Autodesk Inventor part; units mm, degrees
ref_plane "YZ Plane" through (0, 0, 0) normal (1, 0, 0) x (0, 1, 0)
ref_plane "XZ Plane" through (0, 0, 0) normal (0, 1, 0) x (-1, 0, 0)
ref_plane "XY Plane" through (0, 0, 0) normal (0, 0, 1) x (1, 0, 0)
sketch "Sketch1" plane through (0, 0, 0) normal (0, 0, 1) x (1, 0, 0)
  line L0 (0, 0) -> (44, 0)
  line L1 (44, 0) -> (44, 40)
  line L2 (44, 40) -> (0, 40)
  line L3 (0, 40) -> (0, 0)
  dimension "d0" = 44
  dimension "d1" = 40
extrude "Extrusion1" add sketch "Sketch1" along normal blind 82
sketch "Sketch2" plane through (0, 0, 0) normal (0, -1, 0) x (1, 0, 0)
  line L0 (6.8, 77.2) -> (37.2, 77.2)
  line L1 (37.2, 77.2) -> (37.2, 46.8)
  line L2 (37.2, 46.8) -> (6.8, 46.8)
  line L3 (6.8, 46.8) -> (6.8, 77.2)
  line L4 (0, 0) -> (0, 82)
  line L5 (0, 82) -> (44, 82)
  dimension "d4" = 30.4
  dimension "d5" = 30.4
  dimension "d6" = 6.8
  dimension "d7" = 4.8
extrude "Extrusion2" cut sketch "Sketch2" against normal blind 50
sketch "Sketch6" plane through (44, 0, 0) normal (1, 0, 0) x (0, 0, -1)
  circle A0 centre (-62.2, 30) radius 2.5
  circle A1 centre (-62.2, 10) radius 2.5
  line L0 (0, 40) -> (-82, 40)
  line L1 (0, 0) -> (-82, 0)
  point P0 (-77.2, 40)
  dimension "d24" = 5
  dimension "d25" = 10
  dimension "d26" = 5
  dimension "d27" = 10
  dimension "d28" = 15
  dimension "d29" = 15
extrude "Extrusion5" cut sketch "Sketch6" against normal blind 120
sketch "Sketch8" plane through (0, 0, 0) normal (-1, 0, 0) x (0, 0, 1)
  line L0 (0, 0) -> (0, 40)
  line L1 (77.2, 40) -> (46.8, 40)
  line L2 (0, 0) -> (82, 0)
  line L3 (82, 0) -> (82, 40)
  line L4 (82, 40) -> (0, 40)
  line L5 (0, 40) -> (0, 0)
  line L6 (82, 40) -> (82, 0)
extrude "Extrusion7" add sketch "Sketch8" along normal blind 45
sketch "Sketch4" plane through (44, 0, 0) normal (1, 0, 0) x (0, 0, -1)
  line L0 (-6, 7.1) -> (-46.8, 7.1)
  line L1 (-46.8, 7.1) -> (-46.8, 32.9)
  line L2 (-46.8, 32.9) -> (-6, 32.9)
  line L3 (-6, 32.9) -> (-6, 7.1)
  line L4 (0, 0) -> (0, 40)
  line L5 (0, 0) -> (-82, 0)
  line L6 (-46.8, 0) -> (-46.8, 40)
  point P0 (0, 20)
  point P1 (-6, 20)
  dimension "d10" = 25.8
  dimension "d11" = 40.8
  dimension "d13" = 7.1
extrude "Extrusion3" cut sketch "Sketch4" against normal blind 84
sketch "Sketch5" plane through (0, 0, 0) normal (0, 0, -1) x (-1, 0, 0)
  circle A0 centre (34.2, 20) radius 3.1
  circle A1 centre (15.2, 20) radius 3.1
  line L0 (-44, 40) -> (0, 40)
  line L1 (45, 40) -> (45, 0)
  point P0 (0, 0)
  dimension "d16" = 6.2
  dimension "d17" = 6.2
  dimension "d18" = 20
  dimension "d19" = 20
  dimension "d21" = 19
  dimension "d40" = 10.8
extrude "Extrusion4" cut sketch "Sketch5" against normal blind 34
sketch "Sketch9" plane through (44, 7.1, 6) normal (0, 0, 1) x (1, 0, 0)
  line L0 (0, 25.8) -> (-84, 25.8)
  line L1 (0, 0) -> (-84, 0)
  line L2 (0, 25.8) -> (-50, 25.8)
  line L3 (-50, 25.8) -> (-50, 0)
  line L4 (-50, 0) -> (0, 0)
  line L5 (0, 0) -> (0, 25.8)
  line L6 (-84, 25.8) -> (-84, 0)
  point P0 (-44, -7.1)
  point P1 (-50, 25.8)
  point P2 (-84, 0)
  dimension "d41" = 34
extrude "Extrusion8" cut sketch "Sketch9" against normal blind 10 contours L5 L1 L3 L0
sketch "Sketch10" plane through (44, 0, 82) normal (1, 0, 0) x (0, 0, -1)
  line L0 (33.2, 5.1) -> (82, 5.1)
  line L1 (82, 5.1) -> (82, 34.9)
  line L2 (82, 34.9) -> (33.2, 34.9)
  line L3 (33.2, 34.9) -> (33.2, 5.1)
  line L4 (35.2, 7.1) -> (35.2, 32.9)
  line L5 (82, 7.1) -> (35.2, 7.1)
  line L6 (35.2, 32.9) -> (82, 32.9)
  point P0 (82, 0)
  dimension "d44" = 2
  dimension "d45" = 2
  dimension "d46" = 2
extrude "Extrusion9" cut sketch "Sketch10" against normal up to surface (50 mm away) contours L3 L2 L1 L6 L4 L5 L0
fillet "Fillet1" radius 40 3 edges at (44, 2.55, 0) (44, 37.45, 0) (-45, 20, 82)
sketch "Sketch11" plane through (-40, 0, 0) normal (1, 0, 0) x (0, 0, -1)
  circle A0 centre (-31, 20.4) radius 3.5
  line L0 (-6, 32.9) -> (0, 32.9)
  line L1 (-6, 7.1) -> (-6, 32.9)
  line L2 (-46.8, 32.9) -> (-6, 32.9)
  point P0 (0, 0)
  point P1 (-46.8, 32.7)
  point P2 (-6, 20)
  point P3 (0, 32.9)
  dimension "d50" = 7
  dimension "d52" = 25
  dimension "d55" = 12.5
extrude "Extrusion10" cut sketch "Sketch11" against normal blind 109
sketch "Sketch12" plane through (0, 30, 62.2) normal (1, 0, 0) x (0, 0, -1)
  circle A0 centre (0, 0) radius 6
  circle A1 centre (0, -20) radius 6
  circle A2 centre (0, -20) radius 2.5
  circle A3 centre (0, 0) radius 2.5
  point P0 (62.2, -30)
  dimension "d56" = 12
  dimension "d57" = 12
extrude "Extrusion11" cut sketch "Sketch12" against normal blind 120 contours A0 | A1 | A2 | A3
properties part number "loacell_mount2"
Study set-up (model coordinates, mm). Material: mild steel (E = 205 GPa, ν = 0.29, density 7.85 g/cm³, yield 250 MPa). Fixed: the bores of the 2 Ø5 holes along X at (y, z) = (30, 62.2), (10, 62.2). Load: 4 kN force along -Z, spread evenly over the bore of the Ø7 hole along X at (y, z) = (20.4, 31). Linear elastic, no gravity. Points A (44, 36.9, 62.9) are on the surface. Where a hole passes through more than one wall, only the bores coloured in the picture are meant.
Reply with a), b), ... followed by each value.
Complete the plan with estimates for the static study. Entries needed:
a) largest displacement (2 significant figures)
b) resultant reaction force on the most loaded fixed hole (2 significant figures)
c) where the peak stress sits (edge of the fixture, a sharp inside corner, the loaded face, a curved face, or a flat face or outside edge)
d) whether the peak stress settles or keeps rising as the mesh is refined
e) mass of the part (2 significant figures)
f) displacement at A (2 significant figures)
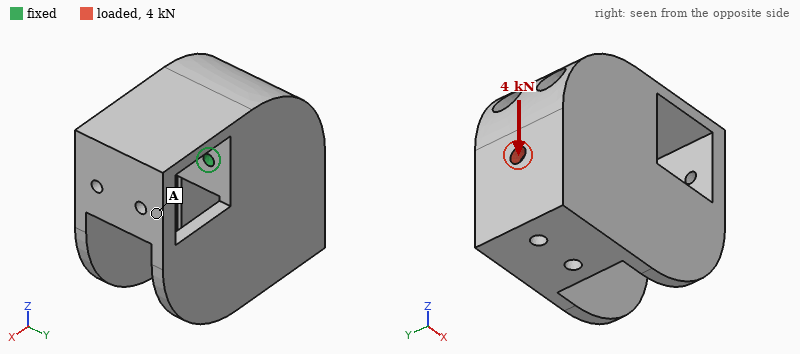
a) 0.19 mm
b) 2.1 kN
c) edge of the fixture
d) keeps rising
e) 950 g
f) 0.096 mm
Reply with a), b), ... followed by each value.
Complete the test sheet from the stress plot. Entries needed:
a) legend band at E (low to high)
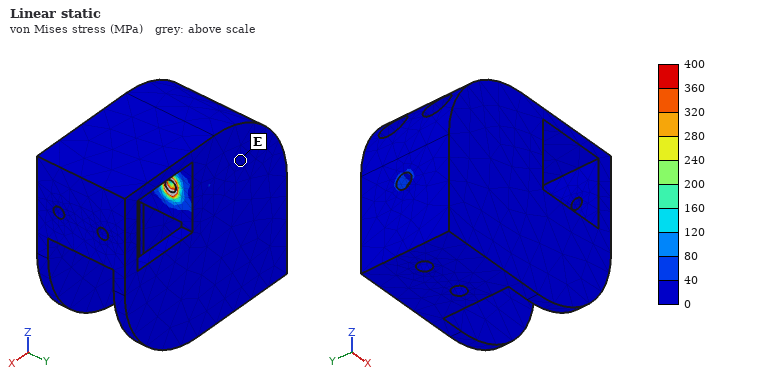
a) 0 to 40 MPa
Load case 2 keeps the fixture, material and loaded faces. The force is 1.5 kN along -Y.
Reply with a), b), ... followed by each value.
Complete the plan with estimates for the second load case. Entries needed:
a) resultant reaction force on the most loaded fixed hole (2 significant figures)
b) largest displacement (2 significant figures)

a) 3.5 kN
b) 21 µm
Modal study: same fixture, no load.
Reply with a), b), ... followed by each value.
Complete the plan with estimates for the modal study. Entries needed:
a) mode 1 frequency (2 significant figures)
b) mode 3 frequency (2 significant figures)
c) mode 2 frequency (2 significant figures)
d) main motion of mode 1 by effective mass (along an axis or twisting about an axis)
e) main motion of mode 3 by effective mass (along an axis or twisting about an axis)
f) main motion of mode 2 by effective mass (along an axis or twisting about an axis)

a) 1100 Hz
b) 2800 Hz
c) 2100 Hz
d) along X
e) twisting about Z
f) along Y
